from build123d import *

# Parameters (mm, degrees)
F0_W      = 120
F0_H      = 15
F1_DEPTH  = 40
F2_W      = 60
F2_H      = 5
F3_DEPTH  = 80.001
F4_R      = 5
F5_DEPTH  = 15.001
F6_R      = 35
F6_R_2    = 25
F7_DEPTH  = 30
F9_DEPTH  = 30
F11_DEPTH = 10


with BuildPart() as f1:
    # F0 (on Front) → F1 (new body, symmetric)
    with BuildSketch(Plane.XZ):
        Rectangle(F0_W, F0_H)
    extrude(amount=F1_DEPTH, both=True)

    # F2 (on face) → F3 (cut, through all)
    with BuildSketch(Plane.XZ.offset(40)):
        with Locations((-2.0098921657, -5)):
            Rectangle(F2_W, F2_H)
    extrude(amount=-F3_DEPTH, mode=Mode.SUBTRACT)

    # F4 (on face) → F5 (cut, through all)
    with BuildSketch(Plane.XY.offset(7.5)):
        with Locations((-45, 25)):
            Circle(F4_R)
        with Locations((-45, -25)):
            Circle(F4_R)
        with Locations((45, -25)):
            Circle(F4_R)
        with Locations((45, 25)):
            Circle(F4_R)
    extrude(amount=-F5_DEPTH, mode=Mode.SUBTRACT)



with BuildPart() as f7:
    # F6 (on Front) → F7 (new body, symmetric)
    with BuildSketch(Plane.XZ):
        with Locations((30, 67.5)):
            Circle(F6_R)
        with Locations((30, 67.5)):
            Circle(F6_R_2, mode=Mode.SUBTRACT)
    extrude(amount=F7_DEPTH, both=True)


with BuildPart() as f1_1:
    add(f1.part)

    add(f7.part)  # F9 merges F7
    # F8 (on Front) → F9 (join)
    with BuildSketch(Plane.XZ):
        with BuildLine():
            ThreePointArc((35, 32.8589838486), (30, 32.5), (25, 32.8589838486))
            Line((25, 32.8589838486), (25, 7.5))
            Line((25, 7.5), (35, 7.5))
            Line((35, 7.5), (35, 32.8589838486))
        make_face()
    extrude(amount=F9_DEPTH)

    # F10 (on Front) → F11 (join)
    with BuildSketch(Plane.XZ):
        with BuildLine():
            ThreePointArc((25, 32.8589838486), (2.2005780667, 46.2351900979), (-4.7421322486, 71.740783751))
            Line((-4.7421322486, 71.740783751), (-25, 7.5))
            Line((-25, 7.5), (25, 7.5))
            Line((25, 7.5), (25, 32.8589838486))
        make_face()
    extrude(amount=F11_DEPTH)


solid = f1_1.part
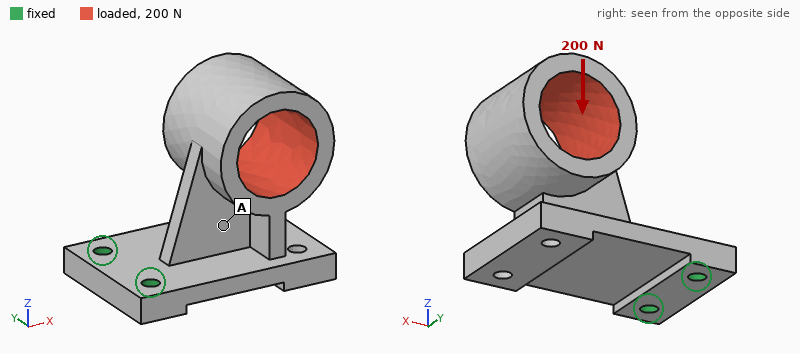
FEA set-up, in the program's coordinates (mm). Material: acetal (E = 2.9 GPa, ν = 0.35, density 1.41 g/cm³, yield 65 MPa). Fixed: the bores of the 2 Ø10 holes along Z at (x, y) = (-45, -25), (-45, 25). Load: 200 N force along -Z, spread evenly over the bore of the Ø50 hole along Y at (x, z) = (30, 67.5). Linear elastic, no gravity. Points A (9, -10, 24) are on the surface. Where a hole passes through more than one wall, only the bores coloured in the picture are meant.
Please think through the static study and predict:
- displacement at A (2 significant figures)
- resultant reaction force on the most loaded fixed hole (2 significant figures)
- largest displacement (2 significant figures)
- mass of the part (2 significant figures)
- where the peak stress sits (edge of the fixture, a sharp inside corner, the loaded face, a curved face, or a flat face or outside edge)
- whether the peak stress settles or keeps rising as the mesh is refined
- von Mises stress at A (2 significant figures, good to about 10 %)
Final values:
0.63 mm
100 N
1.9 mm
360 g
edge of the fixture
keeps rising
0.67 MPa
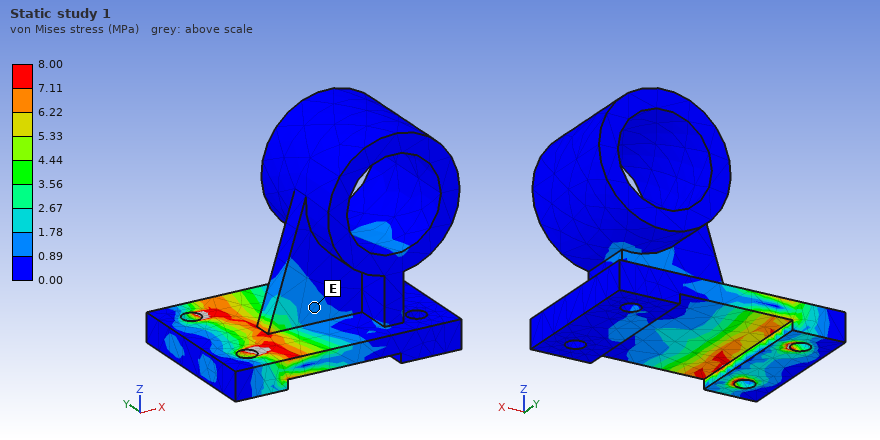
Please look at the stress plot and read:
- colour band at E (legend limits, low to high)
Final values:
0.89 to 1.78 MPa
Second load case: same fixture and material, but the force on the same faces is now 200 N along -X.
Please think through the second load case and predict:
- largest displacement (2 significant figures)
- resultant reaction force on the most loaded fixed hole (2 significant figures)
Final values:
2.2 mm
110 N
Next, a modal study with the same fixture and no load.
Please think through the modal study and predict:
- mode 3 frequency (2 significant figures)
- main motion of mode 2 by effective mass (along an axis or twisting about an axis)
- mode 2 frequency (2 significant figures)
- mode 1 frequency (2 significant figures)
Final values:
510 Hz
along Y
150 Hz
100 Hz
